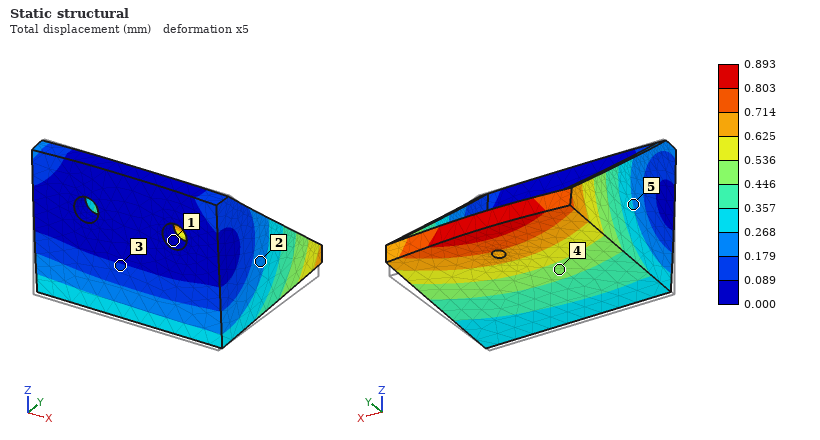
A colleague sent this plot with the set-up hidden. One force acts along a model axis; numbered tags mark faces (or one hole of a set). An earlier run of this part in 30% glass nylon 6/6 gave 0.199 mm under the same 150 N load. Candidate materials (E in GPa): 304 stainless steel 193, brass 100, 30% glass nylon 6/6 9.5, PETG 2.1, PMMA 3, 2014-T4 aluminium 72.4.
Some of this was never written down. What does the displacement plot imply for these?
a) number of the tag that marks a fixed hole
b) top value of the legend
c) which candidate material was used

1
0.893 mm
PETG
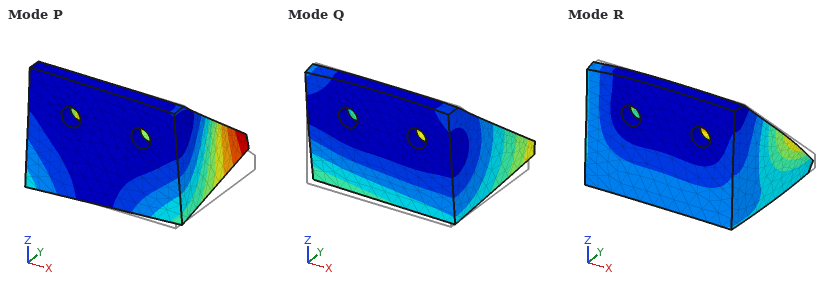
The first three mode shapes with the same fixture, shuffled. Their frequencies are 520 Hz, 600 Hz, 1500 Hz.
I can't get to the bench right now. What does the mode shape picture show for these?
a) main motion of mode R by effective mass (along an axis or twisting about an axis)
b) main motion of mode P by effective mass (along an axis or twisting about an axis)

along Y
along X
